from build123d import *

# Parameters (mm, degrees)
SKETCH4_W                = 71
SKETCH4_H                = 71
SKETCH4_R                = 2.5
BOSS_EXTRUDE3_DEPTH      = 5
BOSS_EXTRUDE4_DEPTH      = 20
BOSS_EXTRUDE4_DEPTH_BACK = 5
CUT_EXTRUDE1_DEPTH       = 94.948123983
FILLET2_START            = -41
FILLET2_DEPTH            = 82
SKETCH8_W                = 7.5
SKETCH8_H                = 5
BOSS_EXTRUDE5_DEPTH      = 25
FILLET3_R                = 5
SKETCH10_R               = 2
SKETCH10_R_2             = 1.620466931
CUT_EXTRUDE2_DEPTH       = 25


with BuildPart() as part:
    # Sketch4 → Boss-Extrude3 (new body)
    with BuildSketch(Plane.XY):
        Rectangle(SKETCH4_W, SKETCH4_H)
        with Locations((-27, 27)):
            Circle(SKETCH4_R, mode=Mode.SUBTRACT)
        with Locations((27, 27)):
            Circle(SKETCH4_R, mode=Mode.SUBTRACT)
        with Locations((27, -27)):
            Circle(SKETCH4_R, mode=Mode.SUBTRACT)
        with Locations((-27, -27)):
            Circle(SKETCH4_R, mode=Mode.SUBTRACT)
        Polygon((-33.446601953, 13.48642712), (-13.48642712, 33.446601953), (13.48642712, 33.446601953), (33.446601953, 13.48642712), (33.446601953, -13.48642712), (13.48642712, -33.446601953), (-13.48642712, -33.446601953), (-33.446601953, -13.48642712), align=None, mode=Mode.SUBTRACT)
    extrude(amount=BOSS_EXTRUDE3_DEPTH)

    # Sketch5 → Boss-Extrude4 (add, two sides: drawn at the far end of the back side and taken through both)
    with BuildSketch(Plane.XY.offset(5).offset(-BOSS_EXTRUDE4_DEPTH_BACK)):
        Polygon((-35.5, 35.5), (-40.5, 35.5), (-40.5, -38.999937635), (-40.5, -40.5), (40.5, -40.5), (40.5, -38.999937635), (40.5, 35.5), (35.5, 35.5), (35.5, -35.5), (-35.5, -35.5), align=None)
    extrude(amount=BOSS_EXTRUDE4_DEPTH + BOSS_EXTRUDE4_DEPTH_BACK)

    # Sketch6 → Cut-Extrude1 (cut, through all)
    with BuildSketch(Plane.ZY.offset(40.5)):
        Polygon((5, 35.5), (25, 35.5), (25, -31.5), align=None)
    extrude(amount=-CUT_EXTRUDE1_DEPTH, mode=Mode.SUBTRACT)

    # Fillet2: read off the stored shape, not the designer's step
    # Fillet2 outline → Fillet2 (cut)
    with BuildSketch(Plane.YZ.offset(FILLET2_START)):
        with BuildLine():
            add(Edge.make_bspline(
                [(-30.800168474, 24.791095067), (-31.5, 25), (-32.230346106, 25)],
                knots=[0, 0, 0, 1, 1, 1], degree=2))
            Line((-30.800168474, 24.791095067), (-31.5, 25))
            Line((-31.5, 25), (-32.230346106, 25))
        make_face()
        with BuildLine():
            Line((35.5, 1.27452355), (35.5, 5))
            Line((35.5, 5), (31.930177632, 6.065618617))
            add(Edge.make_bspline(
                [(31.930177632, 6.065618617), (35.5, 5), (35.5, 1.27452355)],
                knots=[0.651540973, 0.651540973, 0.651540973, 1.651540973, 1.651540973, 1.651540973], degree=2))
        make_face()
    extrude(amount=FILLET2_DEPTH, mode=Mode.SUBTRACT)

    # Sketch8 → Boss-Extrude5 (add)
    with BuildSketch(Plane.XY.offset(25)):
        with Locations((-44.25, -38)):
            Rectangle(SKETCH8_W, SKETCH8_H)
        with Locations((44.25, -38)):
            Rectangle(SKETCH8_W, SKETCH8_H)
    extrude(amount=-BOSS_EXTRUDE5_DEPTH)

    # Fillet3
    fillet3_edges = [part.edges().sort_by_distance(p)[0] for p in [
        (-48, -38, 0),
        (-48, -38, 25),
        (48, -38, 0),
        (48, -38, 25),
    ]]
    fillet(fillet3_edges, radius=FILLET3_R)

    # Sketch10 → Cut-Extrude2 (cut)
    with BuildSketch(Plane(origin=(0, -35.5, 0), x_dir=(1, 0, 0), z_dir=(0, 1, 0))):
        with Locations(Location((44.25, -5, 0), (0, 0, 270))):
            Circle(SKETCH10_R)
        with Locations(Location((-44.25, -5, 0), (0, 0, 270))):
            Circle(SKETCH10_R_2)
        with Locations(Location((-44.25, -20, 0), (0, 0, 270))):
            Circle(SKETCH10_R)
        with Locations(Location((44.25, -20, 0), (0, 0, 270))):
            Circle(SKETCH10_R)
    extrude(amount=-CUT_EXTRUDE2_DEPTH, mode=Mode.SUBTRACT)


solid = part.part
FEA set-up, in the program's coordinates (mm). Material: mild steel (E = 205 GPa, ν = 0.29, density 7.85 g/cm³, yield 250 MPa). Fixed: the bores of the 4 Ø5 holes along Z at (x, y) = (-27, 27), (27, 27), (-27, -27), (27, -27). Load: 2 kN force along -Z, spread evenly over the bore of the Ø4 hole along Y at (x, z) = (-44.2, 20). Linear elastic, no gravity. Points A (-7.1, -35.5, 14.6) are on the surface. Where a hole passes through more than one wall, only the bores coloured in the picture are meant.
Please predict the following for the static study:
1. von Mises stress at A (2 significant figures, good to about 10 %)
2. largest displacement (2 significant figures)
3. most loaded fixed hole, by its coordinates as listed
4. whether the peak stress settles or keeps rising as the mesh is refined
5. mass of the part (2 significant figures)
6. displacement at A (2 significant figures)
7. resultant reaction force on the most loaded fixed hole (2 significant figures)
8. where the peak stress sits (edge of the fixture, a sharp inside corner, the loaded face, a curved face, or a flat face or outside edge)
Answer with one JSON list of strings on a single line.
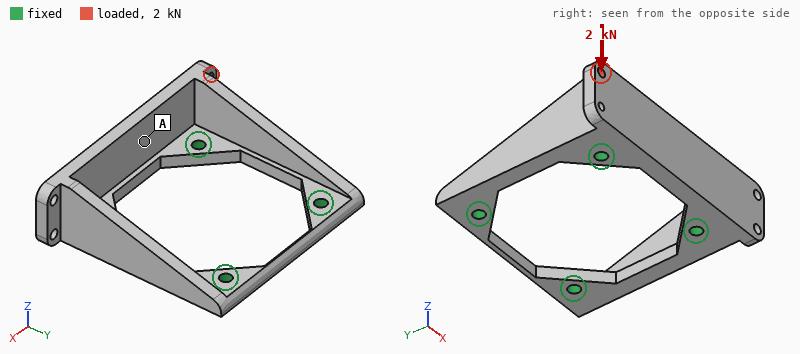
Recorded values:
["17 MPa", "32 µm", "(-27, -27)", "keeps rising", "230 g", "6.9 µm", "2.8 kN", "edge of the fixture"]
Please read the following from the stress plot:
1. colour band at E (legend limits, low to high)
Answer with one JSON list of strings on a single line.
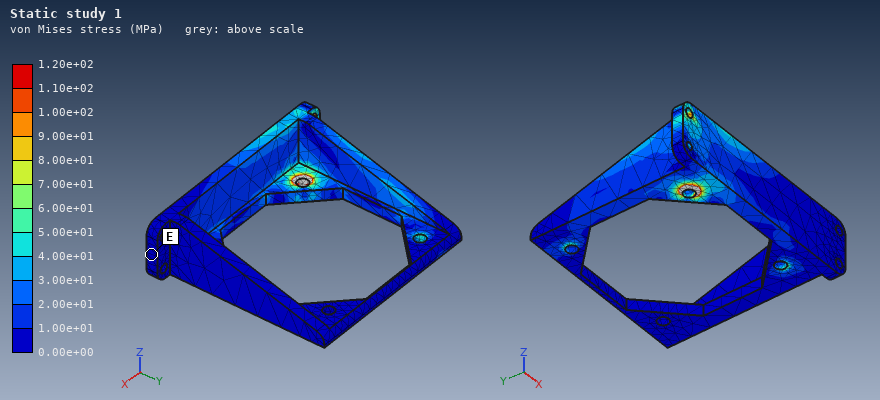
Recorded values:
["0.00e+00 to 1.00e+01 MPa"]
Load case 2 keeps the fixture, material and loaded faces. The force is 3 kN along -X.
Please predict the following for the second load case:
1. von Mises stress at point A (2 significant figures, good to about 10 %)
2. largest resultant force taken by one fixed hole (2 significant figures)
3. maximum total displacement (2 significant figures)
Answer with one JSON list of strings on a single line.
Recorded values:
["22 MPa", "1.8 kN", "26 µm"]
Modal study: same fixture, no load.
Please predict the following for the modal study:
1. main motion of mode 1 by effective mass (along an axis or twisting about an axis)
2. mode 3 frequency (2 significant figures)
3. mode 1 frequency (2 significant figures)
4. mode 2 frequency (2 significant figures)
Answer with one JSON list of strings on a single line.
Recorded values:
["along Y", "7800 Hz", "5600 Hz", "7500 Hz"]
